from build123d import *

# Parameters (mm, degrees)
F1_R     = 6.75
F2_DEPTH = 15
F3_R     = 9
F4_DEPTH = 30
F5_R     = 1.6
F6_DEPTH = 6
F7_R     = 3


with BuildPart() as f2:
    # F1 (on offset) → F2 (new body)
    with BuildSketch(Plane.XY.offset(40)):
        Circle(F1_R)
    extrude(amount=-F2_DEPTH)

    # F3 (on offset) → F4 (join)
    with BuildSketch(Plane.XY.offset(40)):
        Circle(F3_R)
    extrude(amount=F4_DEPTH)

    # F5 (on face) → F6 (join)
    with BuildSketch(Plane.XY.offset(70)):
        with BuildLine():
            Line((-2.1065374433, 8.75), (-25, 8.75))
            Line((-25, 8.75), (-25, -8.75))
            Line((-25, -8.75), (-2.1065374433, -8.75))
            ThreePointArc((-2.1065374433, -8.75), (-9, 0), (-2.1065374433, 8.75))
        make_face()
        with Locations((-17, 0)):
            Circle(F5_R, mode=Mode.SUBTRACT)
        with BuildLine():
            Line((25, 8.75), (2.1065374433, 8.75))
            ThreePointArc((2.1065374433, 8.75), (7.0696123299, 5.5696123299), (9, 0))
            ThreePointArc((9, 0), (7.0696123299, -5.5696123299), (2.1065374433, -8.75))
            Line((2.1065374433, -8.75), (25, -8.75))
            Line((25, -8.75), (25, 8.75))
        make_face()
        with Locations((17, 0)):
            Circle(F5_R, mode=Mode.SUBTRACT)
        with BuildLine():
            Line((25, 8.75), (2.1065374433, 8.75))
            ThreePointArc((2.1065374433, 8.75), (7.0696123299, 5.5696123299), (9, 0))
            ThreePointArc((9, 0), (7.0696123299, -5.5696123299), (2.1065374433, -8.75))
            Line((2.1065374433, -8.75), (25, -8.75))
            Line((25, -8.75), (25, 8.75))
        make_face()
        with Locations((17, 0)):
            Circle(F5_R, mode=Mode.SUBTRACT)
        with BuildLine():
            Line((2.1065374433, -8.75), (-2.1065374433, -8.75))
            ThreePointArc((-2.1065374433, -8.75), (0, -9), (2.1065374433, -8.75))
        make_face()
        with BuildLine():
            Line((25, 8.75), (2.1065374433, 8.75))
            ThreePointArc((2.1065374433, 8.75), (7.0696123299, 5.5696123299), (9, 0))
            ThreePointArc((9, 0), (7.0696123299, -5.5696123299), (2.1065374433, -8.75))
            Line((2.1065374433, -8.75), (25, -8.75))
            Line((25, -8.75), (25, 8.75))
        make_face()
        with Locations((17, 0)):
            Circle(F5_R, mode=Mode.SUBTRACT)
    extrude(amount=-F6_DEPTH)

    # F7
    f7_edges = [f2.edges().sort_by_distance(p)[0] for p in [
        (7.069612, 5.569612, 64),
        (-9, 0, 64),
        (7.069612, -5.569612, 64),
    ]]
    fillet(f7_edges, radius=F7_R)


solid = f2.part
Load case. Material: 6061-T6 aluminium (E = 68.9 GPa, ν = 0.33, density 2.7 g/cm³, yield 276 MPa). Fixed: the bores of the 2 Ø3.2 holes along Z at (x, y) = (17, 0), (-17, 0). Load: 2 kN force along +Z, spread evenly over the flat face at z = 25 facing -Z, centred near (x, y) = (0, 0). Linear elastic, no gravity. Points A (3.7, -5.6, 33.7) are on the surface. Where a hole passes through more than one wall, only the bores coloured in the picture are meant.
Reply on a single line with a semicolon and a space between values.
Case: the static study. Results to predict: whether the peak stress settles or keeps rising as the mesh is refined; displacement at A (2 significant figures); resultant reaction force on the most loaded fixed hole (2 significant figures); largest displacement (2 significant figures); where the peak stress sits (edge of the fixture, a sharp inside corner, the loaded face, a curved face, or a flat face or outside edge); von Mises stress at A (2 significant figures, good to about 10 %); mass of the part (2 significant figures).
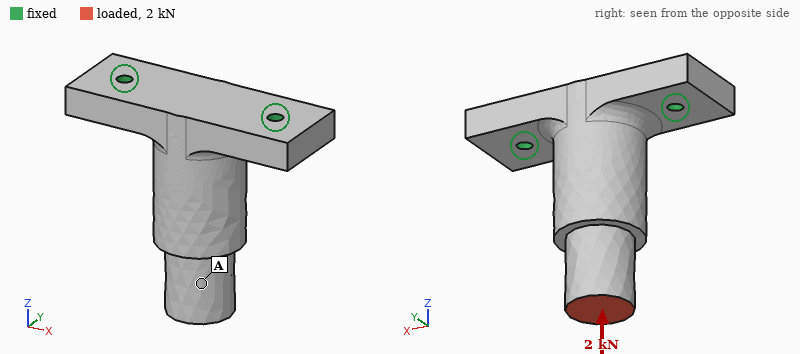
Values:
keeps rising; 15 µm; 1.1 kN; 17 µm; edge of the fixture; 14 MPa; 36 g
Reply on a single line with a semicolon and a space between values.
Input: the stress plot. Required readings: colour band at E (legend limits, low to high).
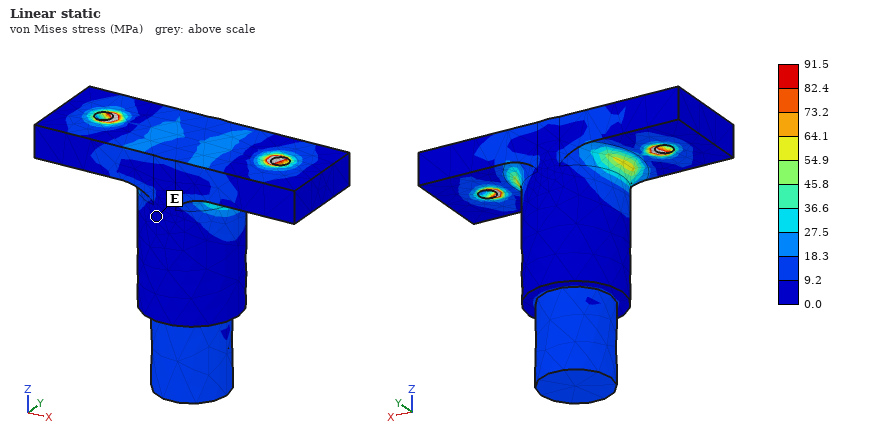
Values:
0.0 to 9.2 MPa
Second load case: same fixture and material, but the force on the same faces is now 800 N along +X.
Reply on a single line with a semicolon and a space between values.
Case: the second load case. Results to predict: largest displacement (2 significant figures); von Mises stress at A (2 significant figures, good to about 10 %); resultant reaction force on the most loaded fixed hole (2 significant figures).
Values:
98 µm; 19 MPa; 1.3 kN
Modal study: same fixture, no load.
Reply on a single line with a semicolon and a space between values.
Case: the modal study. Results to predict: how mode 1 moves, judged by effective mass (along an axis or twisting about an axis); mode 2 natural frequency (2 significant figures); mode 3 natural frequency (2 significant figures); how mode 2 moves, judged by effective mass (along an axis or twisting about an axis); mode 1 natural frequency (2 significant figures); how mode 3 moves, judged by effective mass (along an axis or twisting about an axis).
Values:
along Y; 6500 Hz; 12 kHz; along X; 3100 Hz; along Z
